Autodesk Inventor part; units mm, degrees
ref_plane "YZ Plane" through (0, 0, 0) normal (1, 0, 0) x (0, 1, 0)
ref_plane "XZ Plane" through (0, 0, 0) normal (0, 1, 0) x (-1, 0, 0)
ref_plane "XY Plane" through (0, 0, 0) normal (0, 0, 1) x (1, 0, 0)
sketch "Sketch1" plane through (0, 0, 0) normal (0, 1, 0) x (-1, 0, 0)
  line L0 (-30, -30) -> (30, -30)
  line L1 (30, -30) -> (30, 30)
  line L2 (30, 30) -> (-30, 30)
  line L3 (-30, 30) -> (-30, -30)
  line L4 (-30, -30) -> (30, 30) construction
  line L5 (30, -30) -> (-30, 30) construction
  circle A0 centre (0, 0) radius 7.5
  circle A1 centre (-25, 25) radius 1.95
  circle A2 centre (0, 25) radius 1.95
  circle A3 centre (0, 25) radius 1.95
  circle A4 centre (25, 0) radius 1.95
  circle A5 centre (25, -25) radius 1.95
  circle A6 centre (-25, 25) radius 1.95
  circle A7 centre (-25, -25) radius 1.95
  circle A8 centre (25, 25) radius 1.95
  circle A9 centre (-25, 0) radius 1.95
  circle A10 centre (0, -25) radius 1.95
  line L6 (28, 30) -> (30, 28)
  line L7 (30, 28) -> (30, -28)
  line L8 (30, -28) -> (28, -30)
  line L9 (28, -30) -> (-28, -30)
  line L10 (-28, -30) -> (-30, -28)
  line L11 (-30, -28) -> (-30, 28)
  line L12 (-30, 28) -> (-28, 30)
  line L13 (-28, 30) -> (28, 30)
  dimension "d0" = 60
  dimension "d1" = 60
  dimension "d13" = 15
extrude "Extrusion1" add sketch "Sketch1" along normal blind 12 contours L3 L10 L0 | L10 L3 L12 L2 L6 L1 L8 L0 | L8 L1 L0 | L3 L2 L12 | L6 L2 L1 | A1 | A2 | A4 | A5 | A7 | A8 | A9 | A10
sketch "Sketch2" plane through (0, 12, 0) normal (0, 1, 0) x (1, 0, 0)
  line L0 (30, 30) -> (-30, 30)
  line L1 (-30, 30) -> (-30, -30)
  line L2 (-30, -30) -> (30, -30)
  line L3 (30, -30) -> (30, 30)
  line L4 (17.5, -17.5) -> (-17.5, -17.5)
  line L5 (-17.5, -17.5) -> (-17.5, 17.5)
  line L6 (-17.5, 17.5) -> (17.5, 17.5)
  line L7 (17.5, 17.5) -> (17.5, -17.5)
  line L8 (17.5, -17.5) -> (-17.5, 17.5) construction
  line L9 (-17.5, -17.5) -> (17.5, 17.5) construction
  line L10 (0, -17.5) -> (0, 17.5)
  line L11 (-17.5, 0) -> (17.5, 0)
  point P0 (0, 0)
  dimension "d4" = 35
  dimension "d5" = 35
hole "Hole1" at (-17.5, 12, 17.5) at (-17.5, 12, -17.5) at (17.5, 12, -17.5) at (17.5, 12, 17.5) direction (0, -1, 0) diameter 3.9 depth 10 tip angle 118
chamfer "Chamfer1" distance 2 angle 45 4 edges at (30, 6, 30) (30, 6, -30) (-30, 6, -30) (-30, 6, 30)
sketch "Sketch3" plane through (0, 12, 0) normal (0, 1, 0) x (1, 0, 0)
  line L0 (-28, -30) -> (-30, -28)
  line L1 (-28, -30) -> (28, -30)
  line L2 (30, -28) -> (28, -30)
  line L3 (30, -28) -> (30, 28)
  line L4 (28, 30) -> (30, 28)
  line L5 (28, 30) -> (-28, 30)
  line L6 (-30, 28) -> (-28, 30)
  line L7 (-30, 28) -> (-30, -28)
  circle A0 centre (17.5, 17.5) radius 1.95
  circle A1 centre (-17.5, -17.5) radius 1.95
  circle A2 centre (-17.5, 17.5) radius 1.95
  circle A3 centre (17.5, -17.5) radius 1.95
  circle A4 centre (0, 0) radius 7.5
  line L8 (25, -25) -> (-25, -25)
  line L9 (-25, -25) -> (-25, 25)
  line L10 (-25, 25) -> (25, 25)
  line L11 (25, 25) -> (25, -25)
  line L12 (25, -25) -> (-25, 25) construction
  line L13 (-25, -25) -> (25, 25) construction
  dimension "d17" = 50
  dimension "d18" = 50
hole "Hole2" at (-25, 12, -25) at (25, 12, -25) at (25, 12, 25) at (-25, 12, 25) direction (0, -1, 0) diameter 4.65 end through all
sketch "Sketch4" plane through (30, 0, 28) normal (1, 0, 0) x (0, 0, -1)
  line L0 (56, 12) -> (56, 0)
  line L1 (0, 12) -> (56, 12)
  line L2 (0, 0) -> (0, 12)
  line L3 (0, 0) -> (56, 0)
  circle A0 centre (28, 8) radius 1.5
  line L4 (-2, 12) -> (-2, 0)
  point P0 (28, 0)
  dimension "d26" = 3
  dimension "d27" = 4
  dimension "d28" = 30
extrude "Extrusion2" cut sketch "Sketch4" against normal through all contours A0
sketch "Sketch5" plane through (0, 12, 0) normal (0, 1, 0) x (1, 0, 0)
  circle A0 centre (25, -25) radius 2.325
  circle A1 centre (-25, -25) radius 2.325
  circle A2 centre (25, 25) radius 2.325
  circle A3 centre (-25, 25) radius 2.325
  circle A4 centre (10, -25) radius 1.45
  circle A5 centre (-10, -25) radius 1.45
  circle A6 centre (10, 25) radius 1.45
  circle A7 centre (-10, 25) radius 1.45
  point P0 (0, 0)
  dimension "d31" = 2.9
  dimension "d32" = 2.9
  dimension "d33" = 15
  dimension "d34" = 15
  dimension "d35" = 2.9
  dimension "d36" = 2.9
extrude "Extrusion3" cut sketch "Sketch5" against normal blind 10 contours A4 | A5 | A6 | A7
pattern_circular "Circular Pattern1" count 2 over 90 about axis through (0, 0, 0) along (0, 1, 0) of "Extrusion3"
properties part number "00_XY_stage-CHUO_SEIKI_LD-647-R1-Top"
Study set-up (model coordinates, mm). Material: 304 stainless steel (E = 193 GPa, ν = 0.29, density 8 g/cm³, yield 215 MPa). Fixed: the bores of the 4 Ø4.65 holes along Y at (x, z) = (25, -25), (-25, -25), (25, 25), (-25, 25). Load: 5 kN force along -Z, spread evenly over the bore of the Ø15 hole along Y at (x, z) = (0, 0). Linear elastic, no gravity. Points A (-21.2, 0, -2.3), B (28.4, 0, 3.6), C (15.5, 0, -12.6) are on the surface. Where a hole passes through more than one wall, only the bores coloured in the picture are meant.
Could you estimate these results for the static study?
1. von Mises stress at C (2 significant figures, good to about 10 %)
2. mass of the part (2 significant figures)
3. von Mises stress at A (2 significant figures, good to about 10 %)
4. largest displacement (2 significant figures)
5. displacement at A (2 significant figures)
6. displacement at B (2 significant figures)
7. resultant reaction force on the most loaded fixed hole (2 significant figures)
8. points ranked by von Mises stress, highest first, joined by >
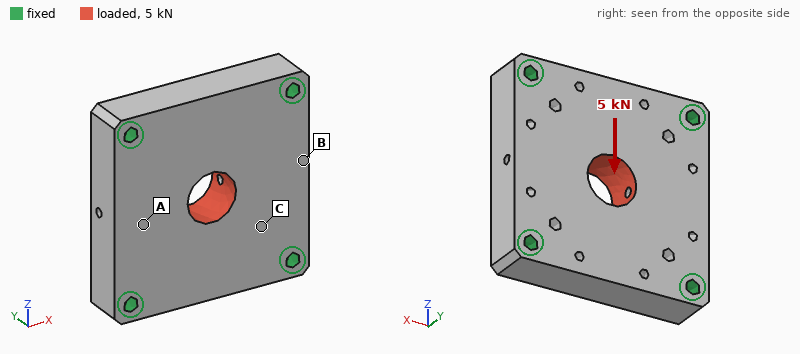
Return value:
7.8 MPa
310 g
4.6 MPa
1.7 µm
0.62 µm
0.42 µm
1.4 kN
C > A > B
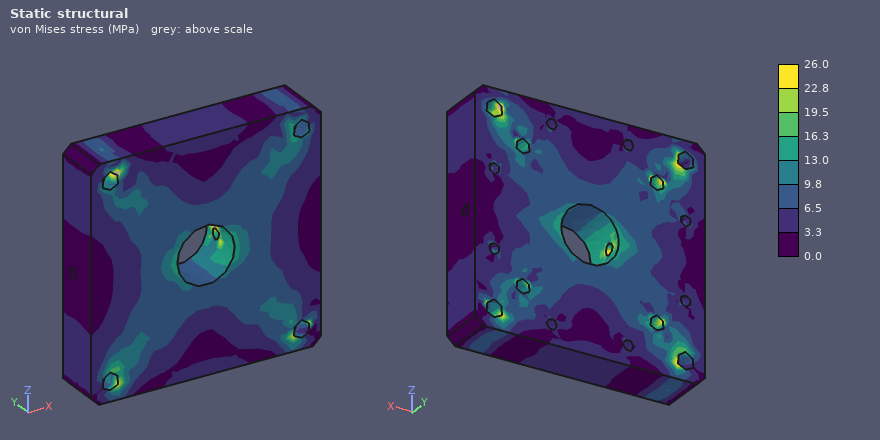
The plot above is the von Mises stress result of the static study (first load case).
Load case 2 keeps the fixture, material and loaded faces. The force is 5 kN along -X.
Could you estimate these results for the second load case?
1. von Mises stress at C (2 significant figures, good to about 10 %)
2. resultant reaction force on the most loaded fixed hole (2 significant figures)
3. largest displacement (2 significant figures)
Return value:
8.4 MPa
1.4 kN
1.7 µm
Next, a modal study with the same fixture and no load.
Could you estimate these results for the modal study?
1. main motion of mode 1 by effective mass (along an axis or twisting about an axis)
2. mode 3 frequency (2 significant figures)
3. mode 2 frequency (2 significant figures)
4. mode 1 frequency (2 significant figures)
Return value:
along Y
20 kHz
19 kHz
13 kHz
